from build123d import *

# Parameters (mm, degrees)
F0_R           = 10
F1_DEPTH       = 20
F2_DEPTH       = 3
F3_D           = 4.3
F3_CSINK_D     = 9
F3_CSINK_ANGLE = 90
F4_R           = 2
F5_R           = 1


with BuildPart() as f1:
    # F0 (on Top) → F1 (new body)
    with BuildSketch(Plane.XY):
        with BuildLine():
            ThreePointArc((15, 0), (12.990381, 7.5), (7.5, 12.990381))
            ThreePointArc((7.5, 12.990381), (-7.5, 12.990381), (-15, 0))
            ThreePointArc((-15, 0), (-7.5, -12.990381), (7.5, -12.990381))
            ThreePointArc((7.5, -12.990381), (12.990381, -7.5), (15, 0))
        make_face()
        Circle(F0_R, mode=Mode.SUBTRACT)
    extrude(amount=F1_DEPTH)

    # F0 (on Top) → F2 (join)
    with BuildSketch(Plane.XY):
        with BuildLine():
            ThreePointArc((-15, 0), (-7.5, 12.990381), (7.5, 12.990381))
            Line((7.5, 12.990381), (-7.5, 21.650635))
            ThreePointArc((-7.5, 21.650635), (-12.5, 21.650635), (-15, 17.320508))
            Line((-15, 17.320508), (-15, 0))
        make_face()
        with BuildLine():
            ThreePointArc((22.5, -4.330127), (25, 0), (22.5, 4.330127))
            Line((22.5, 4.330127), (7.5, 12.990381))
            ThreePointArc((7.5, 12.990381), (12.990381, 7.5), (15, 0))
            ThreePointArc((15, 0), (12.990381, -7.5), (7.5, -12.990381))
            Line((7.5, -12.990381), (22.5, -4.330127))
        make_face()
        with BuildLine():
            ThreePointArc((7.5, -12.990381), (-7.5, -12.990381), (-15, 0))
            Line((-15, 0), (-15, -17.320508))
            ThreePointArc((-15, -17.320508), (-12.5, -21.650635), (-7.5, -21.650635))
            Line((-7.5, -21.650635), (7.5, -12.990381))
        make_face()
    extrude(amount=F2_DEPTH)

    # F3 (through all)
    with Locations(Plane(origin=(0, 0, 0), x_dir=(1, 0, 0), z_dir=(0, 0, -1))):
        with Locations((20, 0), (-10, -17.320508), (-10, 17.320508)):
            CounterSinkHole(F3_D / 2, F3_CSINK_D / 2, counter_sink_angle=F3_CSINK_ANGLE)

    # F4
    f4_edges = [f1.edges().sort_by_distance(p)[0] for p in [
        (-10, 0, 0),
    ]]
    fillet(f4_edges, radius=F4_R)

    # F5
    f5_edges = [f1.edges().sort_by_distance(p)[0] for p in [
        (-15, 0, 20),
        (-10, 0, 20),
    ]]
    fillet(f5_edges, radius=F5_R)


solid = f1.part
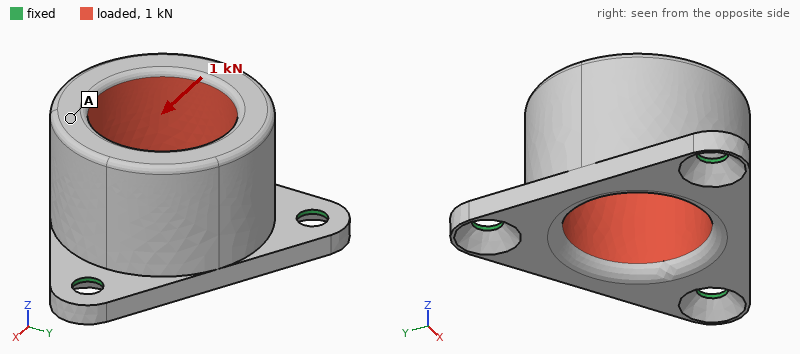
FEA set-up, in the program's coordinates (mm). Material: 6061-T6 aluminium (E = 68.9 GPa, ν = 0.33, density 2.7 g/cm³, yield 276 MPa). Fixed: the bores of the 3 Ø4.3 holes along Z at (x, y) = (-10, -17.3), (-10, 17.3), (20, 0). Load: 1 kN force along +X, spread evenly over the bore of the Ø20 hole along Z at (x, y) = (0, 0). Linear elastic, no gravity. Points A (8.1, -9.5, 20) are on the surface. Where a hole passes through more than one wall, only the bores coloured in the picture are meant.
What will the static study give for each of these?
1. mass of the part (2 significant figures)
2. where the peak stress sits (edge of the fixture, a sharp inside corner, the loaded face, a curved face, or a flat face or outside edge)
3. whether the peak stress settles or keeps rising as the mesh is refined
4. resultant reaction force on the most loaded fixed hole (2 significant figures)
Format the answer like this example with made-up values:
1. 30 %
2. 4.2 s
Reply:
1. 24 g
2. edge of the fixture
3. keeps rising
4. 420 N
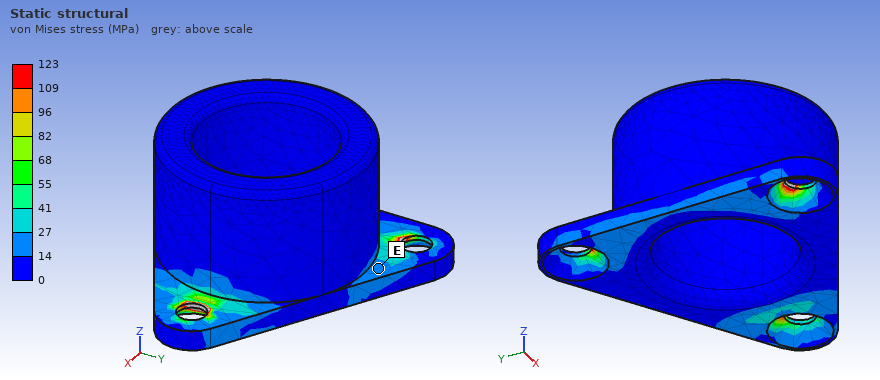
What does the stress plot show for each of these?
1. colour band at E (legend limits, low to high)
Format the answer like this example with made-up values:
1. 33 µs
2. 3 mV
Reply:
1. 14 to 27 MPa
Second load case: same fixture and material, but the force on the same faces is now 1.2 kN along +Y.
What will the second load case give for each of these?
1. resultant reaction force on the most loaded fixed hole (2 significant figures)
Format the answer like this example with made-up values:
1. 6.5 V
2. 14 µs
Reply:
1. 490 N
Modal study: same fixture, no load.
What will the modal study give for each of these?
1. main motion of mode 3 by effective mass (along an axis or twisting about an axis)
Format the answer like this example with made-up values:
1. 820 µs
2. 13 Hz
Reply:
1. along Z
